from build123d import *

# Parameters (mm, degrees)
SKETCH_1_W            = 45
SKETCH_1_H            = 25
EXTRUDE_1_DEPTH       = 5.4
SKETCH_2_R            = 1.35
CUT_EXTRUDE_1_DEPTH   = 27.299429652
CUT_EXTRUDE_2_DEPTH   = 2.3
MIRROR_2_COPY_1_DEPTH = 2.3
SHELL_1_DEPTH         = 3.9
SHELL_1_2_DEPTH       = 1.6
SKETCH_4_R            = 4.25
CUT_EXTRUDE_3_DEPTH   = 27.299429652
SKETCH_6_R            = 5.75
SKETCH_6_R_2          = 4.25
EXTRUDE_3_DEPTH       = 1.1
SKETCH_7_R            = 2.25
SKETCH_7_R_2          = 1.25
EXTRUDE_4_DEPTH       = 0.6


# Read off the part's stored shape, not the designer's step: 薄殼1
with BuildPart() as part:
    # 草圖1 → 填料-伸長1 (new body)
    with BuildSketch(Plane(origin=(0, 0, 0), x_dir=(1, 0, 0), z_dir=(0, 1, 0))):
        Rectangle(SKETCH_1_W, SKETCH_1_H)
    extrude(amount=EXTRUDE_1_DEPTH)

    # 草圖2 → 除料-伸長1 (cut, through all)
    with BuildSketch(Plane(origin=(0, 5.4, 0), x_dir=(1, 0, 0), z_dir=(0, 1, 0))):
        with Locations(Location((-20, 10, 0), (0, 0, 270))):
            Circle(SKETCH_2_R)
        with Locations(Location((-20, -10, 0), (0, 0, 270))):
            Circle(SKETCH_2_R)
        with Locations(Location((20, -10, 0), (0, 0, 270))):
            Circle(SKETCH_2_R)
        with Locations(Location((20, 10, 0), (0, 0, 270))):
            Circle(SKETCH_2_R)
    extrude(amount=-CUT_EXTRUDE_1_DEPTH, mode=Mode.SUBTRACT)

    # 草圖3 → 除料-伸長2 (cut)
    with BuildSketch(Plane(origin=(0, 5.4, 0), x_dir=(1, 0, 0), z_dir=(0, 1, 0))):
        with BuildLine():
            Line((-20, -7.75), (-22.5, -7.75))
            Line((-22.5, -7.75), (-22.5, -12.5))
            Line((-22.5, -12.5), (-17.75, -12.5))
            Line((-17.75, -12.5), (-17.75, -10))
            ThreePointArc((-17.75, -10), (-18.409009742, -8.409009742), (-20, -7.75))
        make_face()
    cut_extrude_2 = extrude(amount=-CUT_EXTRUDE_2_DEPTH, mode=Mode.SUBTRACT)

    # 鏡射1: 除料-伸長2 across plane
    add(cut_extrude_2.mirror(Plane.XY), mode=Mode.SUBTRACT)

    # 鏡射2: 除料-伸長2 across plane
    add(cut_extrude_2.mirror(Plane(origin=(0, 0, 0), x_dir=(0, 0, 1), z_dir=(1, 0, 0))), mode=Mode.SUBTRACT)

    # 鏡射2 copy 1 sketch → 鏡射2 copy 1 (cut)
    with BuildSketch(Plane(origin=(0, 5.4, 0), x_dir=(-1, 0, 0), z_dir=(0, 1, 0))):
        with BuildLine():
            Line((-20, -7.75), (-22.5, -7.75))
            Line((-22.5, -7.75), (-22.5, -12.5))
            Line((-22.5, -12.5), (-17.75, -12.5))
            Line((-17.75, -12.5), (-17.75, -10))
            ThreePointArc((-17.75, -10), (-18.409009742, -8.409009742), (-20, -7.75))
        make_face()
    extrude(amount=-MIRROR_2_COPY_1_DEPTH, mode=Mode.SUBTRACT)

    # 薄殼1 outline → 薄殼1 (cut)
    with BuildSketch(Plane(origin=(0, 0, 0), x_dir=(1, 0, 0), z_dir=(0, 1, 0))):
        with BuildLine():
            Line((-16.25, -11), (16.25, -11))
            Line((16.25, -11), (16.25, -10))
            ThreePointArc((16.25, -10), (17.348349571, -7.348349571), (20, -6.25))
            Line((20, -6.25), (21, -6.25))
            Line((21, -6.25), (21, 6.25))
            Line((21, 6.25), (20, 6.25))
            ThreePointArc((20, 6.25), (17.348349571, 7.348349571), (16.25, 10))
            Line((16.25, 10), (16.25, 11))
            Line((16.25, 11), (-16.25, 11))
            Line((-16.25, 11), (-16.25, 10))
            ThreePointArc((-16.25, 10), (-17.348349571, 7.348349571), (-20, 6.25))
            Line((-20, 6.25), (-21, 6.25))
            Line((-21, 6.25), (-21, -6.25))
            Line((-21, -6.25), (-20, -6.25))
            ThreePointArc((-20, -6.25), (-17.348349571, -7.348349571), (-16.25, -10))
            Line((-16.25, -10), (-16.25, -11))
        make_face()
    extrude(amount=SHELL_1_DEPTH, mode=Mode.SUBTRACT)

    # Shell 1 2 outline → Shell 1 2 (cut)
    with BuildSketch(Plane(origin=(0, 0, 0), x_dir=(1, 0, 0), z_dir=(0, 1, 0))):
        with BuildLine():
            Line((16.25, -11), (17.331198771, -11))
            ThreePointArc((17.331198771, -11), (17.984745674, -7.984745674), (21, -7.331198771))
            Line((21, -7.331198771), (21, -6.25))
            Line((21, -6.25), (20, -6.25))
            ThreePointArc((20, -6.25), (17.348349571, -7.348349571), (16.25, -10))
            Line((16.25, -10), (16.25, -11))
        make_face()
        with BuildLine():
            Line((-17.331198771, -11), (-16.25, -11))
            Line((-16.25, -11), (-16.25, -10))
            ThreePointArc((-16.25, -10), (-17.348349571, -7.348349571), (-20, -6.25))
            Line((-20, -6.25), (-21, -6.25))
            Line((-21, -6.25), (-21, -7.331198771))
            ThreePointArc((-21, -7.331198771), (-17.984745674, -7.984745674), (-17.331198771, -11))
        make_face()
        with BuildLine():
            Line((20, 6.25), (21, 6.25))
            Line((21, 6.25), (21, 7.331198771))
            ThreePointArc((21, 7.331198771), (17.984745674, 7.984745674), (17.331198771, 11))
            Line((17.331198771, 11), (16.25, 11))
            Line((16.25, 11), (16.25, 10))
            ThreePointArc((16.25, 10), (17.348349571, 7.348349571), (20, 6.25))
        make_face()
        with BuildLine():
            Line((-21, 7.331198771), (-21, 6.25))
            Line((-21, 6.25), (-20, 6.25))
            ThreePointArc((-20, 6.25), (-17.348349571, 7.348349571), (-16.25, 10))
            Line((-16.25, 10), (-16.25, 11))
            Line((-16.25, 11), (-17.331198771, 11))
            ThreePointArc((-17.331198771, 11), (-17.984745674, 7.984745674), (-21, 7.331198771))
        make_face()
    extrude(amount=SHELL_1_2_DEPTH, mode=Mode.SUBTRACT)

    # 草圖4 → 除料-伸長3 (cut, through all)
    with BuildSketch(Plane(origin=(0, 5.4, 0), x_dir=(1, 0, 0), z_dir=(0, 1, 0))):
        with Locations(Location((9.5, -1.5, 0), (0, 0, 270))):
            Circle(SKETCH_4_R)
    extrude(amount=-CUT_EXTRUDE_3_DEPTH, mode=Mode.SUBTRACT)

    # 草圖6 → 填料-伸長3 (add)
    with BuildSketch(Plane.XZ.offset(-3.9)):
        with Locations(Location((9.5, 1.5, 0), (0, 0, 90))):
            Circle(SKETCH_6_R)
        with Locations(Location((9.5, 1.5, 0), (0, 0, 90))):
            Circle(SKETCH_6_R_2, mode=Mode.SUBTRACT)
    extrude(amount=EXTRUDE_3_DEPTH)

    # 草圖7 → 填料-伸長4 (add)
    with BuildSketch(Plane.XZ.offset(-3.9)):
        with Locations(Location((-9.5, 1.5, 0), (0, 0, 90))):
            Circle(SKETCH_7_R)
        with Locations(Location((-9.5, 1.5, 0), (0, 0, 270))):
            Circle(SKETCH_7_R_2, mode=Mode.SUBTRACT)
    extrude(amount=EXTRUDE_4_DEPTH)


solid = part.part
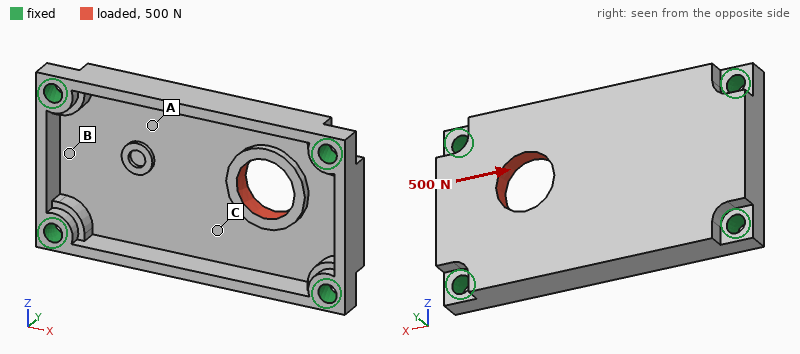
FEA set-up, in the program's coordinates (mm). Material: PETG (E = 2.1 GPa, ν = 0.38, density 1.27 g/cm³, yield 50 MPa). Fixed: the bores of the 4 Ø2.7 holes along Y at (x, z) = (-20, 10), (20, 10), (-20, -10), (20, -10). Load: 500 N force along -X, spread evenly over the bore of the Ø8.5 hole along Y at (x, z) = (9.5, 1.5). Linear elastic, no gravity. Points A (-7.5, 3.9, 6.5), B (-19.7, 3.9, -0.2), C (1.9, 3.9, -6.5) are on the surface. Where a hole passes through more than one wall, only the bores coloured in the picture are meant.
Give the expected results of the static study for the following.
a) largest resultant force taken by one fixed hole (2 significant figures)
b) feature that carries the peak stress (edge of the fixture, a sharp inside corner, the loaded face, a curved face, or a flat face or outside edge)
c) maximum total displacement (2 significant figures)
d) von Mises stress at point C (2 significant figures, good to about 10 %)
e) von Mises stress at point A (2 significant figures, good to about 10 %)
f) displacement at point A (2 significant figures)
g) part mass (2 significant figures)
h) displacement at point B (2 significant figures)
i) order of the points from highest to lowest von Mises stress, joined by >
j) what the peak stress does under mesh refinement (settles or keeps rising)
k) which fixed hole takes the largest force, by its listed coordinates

170 N
edge of the fixture
0.17 mm
9.5 MPa
4.7 MPa
0.080 mm
3.1 g
0.039 mm
C > A > B
keeps rising
(20, 10)
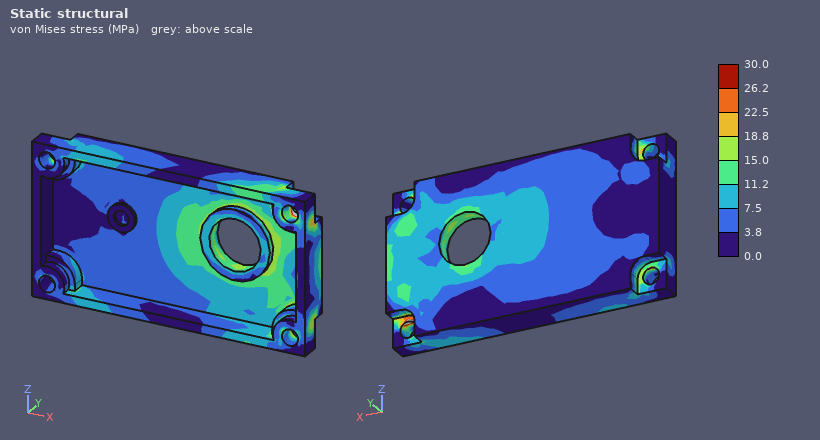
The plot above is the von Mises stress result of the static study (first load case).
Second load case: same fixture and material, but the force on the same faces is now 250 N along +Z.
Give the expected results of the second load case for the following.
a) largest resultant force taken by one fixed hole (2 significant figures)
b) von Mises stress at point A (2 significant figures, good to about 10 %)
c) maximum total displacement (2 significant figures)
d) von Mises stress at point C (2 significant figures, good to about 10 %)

91 N
4.9 MPa
0.17 mm
5.1 MPa
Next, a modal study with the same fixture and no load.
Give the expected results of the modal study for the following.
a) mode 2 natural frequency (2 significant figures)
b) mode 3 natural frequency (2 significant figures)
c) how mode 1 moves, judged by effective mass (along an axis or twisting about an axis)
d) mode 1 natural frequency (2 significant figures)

3400 Hz
4700 Hz
along Y
2400 Hz
